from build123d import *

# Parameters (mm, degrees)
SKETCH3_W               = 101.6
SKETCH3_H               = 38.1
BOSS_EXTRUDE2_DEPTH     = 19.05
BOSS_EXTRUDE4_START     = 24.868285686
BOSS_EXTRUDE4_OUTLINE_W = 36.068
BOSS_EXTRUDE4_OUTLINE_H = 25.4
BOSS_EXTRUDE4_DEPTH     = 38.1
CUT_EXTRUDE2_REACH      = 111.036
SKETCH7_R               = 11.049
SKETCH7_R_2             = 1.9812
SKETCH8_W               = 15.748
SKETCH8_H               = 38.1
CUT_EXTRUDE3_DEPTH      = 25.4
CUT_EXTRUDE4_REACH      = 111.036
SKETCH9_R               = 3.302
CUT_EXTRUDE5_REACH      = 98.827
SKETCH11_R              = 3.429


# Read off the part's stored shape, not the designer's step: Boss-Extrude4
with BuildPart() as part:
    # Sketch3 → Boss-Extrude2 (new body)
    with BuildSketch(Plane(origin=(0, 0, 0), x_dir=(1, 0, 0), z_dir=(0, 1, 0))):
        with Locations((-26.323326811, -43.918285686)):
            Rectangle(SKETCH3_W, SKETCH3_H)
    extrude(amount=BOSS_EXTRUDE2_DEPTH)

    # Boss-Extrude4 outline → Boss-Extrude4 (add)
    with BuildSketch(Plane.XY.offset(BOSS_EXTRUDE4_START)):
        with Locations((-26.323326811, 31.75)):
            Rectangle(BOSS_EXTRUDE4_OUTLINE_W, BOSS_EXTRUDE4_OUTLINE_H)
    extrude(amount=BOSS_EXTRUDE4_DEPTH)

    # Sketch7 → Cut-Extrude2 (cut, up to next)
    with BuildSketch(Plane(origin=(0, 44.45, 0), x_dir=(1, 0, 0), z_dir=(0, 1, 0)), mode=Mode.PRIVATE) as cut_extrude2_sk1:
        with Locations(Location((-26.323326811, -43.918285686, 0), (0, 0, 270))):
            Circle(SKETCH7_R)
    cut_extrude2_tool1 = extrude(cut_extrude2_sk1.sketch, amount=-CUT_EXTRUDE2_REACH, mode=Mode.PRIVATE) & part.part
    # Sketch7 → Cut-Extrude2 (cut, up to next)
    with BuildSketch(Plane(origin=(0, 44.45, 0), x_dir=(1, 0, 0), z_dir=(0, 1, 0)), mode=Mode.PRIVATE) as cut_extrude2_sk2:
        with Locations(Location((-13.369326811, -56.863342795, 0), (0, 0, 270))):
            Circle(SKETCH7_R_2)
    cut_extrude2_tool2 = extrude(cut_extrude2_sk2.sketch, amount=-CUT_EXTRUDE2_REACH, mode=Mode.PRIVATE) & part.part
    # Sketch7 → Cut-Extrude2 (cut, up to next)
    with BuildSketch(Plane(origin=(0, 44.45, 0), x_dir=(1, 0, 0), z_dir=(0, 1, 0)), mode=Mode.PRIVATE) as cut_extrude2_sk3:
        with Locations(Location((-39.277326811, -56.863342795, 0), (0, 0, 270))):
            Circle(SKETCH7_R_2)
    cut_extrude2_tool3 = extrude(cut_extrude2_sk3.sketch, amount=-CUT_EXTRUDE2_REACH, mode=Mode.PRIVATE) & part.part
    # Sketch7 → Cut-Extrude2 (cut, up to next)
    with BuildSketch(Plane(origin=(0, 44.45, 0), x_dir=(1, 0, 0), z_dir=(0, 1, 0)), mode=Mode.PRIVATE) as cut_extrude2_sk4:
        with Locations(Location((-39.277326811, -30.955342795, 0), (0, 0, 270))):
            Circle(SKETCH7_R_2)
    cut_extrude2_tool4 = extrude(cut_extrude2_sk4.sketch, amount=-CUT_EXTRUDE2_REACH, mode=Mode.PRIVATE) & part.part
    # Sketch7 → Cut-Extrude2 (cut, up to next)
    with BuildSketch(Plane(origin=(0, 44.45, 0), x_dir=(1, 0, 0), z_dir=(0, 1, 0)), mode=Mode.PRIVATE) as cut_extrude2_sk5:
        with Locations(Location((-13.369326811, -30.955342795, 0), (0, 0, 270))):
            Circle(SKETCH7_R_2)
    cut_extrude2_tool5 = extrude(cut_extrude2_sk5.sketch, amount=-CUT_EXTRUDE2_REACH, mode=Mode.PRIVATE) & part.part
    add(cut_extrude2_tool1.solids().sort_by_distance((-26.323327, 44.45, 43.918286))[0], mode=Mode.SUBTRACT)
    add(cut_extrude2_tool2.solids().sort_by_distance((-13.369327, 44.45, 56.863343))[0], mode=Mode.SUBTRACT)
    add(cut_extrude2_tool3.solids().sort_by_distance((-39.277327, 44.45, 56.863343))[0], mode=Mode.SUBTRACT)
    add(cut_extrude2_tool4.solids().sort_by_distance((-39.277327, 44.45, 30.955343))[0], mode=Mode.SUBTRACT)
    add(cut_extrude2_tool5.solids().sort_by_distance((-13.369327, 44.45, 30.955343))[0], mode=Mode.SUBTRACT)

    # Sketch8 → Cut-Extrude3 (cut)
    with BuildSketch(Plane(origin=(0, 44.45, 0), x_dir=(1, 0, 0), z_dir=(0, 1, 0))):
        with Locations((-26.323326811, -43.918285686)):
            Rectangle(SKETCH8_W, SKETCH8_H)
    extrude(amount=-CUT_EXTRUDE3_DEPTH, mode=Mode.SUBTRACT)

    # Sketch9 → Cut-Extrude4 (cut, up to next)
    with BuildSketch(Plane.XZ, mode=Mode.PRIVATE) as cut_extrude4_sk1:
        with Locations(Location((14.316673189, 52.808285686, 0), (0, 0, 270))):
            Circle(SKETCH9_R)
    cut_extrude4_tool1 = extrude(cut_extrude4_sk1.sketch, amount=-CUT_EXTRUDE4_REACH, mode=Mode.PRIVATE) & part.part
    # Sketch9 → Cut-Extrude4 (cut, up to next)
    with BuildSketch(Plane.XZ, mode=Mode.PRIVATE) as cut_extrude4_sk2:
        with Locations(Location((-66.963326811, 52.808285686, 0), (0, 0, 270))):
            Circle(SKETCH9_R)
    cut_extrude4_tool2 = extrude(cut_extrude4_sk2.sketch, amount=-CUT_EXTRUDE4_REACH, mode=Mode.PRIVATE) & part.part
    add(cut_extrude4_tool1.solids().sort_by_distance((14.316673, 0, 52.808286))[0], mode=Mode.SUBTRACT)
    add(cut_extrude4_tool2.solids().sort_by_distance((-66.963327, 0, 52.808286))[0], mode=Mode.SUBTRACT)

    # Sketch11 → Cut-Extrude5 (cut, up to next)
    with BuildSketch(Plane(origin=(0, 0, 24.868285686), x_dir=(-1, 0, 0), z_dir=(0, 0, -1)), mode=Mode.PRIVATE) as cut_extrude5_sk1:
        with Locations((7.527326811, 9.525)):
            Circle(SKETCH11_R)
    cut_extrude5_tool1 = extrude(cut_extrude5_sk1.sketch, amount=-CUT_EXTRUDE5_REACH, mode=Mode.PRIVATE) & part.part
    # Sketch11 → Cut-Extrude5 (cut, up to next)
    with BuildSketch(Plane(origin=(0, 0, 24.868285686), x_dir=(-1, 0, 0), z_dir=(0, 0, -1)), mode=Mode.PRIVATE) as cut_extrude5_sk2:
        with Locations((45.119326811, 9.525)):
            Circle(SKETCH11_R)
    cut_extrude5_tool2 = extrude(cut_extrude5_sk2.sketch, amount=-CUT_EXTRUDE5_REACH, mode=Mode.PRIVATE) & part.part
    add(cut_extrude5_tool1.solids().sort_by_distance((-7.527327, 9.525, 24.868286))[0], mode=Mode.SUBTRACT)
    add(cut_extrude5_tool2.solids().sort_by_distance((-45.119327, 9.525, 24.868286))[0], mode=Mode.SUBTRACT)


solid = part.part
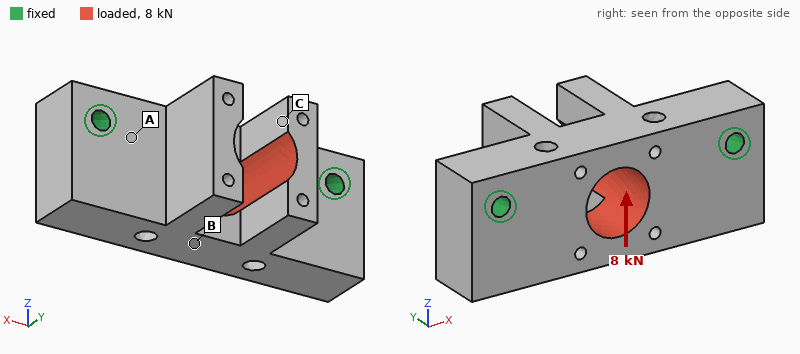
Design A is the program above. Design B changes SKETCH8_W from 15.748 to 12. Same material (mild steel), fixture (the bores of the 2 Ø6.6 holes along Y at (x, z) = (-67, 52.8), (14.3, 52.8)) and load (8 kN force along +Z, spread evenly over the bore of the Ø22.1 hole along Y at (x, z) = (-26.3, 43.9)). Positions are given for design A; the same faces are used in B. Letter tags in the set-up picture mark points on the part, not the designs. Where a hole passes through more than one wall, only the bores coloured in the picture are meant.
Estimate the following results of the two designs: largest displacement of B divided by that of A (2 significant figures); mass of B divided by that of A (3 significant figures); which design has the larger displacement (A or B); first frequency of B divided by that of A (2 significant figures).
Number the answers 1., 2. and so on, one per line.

1. 1.1
2. 1.03
3. B
4. 0.97
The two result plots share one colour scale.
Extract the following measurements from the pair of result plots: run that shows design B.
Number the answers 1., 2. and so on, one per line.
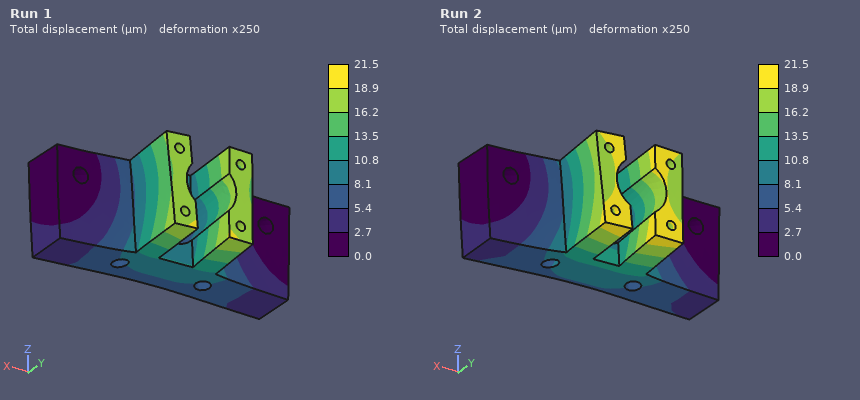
1. Run 2
